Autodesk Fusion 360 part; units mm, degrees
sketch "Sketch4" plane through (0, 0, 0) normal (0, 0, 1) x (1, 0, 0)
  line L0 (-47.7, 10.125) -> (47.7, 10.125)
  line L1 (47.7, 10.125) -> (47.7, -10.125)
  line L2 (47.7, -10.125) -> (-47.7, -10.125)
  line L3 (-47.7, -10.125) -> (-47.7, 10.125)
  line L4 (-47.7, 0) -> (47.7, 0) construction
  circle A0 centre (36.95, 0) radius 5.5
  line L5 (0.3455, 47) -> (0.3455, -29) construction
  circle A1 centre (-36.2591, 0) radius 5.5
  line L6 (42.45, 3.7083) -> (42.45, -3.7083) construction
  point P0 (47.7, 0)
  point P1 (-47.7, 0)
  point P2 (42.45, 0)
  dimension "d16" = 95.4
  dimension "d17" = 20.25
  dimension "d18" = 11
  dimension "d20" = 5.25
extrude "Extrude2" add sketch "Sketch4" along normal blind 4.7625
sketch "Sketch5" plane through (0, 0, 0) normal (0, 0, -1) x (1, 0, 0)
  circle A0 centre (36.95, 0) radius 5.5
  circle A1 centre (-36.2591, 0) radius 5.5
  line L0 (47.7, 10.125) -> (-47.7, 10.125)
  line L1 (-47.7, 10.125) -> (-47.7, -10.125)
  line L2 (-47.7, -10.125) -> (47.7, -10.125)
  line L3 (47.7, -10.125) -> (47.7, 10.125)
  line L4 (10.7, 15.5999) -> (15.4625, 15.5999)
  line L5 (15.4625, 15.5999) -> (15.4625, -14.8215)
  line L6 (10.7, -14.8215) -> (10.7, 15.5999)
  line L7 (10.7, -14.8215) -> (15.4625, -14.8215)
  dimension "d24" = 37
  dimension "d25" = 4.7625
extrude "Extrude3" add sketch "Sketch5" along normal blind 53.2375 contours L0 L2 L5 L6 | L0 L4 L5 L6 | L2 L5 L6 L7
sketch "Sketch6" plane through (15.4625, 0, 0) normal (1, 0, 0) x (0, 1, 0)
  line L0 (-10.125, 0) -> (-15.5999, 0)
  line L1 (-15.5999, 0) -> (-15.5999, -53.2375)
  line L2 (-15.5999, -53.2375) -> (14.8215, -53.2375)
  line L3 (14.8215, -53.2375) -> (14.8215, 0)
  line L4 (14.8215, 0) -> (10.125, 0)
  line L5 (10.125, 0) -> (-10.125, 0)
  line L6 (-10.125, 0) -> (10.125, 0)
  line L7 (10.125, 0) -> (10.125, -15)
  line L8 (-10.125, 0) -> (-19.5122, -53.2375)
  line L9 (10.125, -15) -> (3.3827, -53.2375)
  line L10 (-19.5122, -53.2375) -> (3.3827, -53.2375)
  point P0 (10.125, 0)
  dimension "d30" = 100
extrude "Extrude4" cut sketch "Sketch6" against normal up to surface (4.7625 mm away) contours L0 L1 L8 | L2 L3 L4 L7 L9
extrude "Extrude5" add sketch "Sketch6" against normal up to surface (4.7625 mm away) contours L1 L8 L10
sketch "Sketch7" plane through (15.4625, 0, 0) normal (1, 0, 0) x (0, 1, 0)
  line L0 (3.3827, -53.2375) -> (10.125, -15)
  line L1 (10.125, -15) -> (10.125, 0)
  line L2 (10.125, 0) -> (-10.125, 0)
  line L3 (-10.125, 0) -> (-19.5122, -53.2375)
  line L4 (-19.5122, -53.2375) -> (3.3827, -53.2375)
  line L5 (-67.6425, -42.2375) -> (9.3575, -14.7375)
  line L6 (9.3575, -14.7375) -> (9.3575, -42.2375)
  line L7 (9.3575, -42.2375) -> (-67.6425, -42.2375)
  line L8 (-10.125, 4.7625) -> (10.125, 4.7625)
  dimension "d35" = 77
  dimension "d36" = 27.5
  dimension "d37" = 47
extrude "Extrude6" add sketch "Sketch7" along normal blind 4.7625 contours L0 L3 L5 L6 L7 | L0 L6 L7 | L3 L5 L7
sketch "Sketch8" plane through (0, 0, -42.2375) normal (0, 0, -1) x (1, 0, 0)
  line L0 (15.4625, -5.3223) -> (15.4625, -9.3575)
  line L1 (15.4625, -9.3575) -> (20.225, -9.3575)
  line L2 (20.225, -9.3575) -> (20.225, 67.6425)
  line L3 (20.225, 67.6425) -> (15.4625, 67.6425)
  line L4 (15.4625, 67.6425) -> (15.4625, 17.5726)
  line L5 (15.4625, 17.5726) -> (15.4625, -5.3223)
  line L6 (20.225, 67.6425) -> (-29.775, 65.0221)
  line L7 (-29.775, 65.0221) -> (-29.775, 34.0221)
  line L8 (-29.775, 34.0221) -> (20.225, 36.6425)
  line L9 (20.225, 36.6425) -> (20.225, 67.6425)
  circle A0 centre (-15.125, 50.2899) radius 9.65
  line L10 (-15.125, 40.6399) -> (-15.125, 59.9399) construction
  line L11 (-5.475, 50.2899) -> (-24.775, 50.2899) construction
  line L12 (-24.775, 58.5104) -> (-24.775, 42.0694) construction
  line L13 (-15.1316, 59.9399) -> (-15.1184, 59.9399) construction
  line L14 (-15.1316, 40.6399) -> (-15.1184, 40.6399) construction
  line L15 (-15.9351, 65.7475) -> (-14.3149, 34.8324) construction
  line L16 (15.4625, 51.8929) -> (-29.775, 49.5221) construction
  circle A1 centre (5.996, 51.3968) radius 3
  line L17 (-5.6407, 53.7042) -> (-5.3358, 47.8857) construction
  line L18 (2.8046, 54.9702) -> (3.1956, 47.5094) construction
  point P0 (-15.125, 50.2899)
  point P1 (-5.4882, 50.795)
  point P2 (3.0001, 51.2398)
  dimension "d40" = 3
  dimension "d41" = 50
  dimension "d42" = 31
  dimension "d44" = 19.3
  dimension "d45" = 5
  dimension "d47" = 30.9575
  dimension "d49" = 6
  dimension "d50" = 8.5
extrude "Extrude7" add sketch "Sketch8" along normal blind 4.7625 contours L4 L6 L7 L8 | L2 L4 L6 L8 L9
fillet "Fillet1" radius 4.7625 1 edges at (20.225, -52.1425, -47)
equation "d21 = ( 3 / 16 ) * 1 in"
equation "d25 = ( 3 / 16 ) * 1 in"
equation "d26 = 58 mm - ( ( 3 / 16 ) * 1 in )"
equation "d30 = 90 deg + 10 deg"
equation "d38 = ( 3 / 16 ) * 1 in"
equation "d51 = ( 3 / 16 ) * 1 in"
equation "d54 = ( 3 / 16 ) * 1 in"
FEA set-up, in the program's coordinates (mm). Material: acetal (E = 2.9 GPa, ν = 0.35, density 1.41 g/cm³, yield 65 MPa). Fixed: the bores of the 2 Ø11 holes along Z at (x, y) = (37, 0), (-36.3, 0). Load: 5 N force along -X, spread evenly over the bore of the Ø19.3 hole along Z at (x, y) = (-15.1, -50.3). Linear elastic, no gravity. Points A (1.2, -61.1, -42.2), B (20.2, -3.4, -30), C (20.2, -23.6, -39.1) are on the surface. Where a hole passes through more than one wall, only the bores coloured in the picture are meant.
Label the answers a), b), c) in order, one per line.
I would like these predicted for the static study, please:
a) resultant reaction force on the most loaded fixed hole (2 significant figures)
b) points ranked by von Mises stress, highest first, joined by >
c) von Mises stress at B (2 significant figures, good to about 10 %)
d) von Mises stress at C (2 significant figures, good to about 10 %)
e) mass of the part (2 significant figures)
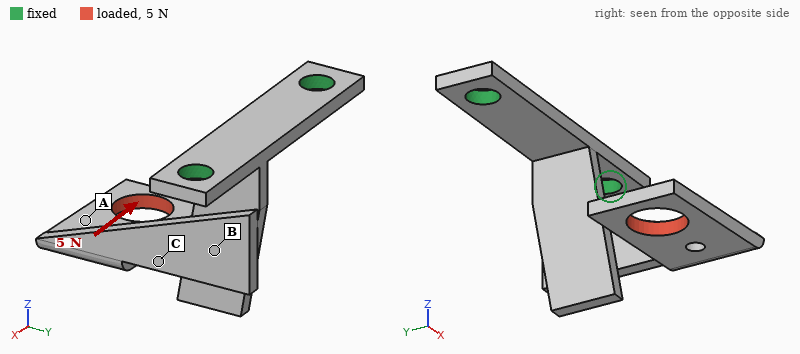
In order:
a) 6.9 N
b) C > B > A
c) 0.86 MPa
d) 2.5 MPa
e) 35 g
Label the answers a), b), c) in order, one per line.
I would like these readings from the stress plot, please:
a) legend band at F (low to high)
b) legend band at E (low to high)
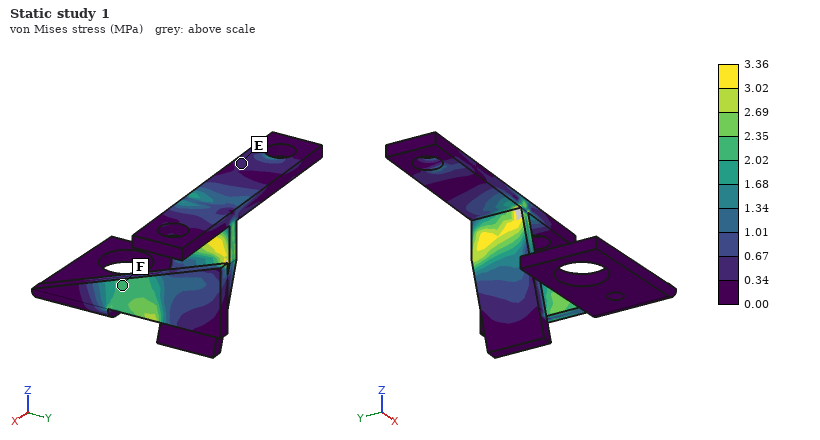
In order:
a) 2.02 to 2.35 MPa
b) 0.34 to 0.67 MPa
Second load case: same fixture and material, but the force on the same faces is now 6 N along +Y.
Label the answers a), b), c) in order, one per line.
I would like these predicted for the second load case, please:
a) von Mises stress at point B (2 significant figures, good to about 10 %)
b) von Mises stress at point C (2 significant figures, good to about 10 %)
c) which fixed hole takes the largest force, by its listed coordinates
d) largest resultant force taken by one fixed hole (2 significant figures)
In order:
a) 0.53 MPa
b) 3.3 MPa
c) (-36.3, 0)
d) 3.9 N
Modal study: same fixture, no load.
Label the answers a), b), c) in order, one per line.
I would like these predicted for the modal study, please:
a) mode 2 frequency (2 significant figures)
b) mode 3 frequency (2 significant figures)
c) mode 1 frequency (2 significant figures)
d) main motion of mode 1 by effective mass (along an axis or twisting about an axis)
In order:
a) 140 Hz
b) 250 Hz
c) 110 Hz
d) along X
